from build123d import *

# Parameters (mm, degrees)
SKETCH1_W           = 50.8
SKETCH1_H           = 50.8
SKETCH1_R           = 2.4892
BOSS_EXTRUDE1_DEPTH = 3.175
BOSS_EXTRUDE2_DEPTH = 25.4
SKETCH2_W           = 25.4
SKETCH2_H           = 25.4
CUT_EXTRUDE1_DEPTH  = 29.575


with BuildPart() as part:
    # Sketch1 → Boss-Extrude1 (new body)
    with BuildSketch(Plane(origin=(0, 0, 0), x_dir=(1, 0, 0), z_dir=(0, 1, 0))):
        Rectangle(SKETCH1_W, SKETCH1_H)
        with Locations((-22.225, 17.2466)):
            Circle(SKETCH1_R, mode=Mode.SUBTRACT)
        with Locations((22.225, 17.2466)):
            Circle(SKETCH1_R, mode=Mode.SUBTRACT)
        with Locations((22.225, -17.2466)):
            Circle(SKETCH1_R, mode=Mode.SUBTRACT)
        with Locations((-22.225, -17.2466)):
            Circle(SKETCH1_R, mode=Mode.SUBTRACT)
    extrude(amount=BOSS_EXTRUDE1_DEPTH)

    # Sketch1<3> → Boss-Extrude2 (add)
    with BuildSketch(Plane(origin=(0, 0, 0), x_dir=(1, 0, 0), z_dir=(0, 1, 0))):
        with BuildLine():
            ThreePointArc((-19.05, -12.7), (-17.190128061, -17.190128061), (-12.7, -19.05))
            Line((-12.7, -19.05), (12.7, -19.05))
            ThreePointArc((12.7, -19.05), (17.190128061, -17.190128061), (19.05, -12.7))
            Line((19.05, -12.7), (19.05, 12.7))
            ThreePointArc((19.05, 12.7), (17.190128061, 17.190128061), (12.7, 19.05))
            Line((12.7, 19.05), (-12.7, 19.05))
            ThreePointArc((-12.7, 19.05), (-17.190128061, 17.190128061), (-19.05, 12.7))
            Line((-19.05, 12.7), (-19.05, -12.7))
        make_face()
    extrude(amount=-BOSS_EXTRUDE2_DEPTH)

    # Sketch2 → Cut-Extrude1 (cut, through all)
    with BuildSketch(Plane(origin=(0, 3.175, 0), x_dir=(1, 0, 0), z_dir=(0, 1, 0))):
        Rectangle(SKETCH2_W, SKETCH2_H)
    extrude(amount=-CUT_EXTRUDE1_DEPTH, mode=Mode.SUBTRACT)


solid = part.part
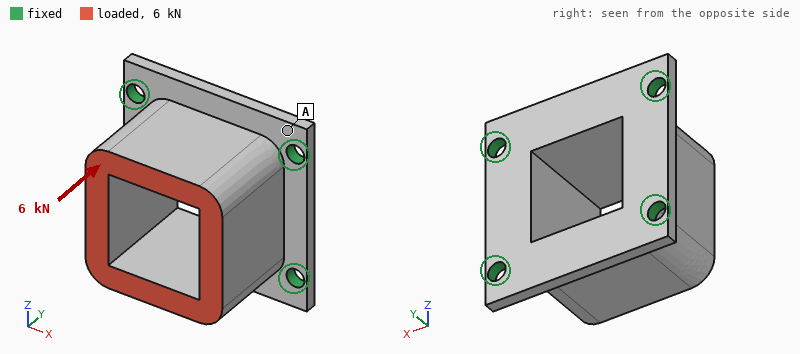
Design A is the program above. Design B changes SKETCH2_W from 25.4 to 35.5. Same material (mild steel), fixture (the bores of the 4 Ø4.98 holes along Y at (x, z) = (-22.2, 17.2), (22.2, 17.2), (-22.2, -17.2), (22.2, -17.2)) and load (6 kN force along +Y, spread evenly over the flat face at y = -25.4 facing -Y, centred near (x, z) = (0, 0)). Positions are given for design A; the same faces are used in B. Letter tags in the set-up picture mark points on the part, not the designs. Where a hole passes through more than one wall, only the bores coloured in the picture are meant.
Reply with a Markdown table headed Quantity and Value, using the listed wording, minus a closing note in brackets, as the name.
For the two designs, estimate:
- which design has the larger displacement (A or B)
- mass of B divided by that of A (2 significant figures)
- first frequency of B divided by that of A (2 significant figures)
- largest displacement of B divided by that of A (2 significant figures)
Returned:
| Quantity | Value |
|---|---|
| which design has the larger displacement | B |
| mass of B divided by that of A | 0.71 |
| first frequency of B divided by that of A | 0.90 |
| largest displacement of B divided by that of A | 1.2 |
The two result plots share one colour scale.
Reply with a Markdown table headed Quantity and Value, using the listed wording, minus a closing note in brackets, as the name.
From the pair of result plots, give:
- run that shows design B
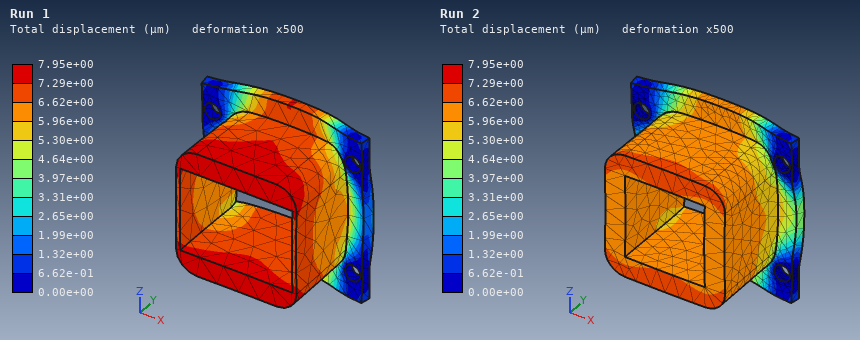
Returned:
| Quantity | Value |
|---|---|
| run that shows design B | Run 1 |
